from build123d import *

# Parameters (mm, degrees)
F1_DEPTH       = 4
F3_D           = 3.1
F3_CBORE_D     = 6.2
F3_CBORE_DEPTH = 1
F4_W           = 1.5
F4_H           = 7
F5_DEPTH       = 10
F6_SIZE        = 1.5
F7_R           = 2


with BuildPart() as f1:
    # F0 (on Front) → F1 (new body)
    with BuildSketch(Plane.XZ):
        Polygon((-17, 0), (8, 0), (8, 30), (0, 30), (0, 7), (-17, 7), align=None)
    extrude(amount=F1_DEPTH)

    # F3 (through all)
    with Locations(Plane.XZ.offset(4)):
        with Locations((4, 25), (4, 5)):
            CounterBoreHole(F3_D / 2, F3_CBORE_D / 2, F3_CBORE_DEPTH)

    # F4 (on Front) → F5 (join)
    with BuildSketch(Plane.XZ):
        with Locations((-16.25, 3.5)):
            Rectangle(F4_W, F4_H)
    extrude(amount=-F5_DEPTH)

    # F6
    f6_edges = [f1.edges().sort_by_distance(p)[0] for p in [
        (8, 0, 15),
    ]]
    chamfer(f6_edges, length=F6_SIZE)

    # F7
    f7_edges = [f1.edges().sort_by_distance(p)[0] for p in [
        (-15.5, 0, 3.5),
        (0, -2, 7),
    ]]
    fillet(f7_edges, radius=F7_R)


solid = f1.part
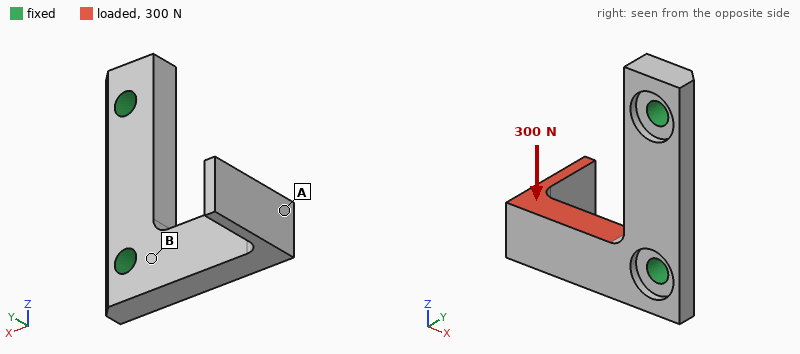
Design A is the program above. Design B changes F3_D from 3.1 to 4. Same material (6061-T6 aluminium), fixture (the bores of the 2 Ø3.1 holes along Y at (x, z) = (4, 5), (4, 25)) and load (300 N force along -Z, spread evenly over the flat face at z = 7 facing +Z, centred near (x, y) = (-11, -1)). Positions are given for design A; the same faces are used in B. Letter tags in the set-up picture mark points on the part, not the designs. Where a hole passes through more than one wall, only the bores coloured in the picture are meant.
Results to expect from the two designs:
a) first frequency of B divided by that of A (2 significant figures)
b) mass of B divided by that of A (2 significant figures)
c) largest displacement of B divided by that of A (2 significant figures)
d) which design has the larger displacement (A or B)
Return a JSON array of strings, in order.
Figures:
["1.1", "0.98", "0.91", "A"]
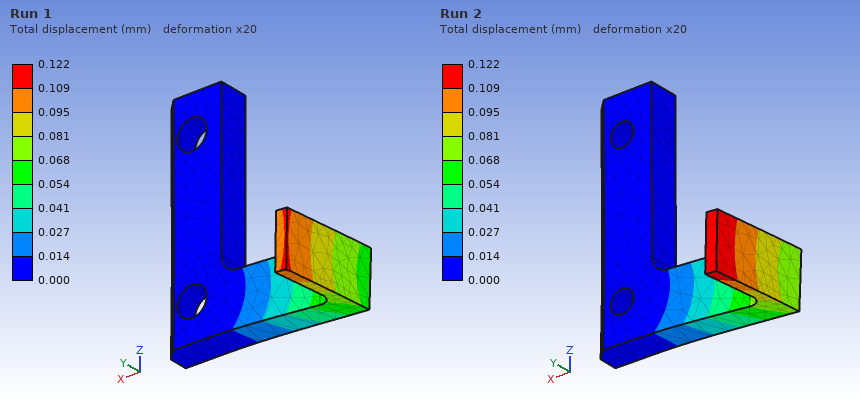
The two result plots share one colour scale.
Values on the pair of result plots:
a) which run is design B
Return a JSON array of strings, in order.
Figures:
["Run 1"]
